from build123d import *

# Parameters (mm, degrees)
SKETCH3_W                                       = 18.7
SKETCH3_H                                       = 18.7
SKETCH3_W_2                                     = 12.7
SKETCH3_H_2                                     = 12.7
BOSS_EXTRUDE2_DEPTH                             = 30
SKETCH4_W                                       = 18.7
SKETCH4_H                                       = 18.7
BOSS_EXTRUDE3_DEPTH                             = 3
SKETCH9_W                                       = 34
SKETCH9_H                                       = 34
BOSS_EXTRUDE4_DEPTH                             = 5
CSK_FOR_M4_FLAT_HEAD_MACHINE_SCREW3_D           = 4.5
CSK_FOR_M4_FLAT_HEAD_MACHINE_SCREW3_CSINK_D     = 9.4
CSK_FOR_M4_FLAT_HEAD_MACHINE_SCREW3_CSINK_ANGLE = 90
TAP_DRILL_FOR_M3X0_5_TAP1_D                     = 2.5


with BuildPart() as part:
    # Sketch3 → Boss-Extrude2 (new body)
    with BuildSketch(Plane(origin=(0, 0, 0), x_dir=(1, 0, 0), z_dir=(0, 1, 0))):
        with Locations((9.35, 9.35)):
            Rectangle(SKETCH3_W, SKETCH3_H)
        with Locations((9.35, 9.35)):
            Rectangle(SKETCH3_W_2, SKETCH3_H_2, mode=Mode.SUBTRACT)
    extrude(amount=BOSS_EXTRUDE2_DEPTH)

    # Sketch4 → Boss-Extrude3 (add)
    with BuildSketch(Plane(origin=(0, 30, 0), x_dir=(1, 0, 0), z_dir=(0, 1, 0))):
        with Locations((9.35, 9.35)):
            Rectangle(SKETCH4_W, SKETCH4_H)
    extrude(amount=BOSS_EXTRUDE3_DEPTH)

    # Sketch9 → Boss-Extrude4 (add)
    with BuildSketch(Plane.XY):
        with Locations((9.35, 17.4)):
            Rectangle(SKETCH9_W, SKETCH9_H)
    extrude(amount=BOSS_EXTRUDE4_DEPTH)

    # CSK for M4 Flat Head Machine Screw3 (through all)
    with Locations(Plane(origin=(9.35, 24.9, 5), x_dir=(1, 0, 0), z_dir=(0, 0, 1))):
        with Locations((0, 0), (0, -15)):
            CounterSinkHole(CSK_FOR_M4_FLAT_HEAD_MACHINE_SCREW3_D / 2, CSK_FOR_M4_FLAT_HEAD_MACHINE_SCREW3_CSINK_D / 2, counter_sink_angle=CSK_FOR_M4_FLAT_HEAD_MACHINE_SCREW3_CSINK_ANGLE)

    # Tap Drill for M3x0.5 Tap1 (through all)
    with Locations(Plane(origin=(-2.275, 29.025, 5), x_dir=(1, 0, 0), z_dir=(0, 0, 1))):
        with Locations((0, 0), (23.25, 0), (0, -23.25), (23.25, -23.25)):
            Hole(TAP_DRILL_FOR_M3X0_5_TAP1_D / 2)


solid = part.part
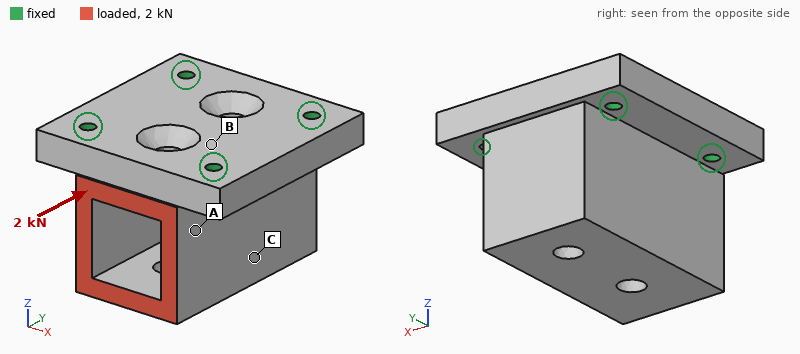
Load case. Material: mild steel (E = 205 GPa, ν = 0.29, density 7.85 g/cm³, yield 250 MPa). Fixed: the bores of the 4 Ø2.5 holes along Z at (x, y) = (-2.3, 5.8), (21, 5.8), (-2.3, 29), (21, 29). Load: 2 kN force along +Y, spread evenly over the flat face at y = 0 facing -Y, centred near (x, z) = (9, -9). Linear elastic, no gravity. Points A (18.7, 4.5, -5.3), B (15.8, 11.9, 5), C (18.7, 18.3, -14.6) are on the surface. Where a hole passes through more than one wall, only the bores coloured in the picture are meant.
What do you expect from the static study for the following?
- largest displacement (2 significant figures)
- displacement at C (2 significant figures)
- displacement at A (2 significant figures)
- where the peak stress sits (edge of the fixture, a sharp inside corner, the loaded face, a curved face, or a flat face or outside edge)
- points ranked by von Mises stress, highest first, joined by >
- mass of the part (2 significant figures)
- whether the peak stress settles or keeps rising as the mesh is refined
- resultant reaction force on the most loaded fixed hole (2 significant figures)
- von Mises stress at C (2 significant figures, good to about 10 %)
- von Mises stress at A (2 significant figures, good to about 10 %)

4.9 µm
2.9 µm
2.2 µm
edge of the fixture
A > C > B
94 g
keeps rising
730 N
10 MPa
17 MPa
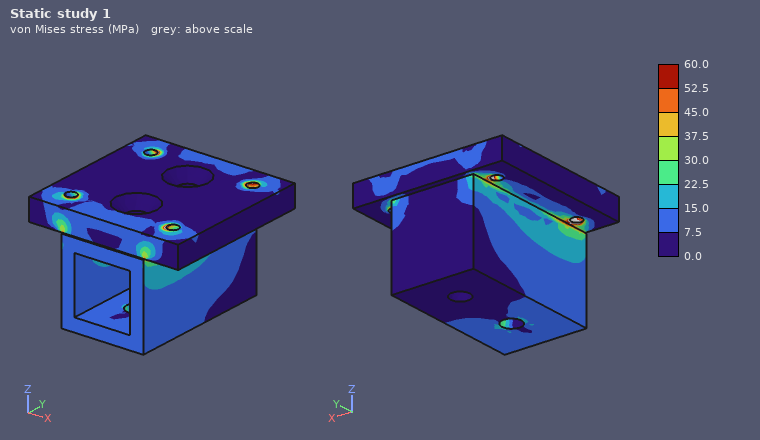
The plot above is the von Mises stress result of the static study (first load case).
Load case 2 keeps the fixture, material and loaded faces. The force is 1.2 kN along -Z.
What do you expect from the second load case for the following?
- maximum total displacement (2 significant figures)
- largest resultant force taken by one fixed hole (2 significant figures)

6.9 µm
750 N
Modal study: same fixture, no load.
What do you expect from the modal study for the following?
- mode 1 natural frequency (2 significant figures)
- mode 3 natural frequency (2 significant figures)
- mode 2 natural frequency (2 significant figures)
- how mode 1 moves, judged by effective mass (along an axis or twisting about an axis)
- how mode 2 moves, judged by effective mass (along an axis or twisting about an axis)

11 kHz
24 kHz
17 kHz
along X
along Y
